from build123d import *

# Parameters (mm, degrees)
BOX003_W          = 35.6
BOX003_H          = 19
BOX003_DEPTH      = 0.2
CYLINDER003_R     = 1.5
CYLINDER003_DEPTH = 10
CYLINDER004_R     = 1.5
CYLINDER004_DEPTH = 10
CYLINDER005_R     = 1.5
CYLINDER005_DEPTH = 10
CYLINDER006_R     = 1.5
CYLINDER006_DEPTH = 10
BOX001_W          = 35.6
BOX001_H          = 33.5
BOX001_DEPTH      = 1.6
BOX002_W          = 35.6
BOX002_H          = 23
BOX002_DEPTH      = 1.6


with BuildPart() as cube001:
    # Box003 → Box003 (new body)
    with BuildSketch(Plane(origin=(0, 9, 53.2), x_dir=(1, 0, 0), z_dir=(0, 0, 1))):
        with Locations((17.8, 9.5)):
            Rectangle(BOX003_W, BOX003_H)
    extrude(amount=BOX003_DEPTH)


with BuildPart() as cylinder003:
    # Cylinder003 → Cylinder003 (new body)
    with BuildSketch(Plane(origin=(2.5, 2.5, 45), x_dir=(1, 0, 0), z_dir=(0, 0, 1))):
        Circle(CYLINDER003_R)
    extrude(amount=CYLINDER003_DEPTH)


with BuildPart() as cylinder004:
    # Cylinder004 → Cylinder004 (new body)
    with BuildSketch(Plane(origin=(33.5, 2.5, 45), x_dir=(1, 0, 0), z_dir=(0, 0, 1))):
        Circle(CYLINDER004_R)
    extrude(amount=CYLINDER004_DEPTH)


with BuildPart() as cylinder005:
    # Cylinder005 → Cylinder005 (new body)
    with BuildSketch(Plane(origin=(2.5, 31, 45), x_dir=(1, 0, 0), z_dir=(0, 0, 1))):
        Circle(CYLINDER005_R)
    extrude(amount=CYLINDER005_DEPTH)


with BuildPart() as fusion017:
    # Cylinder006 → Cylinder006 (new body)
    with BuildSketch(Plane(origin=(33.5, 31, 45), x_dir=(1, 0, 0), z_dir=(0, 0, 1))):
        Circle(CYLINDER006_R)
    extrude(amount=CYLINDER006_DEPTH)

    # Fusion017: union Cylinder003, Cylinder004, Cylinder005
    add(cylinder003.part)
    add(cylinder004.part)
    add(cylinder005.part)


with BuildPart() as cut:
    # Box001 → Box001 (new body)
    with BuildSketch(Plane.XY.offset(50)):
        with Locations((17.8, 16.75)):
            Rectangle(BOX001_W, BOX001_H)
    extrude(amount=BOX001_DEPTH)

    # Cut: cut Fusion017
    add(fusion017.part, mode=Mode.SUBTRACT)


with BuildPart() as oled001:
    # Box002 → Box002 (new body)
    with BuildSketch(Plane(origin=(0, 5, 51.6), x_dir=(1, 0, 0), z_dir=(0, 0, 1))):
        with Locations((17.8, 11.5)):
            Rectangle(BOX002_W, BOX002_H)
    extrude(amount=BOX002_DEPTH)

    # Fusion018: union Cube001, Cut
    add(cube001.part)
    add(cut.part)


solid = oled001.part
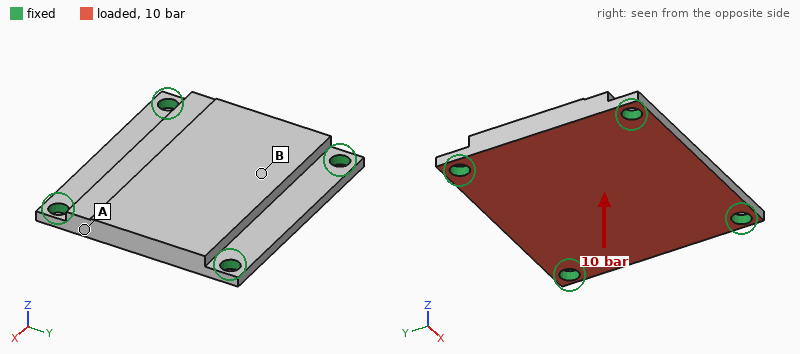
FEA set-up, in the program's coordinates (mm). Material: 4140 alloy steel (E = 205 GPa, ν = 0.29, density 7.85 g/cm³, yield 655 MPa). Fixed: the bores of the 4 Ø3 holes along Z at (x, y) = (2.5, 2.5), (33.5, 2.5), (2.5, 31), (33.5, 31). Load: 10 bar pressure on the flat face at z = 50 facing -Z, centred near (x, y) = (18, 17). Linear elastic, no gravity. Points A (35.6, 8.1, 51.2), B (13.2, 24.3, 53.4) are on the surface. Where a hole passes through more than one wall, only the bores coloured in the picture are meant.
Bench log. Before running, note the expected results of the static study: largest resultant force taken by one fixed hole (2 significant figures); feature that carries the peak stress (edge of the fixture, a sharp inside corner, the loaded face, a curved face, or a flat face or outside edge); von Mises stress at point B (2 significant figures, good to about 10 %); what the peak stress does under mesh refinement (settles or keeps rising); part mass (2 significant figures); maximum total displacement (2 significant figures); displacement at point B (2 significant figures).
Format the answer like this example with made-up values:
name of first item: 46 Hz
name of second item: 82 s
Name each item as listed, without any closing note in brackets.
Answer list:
largest resultant force taken by one fixed hole: 440 N
feature that carries the peak stress: edge of the fixture
von Mises stress at point B: 46 MPa
what the peak stress does under mesh refinement: keeps rising
part mass: 26 g
maximum total displacement: 17 µm
displacement at point B: 14 µm
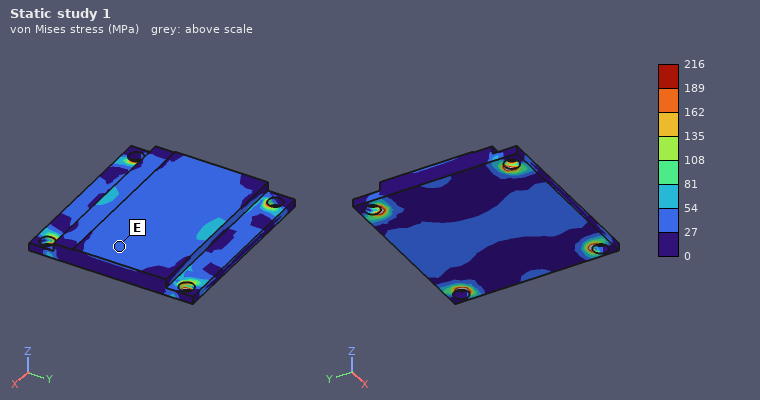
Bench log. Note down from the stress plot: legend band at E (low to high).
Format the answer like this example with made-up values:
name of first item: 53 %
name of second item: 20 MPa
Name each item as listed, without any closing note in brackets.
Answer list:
legend band at E: 27 to 54 MPa
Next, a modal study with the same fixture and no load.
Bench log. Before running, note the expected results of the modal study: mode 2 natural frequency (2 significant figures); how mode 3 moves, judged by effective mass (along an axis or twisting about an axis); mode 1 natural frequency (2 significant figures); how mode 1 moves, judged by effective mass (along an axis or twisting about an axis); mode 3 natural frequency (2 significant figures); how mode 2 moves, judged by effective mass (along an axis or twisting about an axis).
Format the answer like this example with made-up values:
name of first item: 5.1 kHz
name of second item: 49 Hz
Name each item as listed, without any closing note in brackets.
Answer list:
mode 2 natural frequency: 15 kHz
how mode 3 moves, judged by effective mass: twisting about Y
mode 1 natural frequency: 9400 Hz
how mode 1 moves, judged by effective mass: along Z
mode 3 natural frequency: 18 kHz
how mode 2 moves, judged by effective mass: twisting about X
